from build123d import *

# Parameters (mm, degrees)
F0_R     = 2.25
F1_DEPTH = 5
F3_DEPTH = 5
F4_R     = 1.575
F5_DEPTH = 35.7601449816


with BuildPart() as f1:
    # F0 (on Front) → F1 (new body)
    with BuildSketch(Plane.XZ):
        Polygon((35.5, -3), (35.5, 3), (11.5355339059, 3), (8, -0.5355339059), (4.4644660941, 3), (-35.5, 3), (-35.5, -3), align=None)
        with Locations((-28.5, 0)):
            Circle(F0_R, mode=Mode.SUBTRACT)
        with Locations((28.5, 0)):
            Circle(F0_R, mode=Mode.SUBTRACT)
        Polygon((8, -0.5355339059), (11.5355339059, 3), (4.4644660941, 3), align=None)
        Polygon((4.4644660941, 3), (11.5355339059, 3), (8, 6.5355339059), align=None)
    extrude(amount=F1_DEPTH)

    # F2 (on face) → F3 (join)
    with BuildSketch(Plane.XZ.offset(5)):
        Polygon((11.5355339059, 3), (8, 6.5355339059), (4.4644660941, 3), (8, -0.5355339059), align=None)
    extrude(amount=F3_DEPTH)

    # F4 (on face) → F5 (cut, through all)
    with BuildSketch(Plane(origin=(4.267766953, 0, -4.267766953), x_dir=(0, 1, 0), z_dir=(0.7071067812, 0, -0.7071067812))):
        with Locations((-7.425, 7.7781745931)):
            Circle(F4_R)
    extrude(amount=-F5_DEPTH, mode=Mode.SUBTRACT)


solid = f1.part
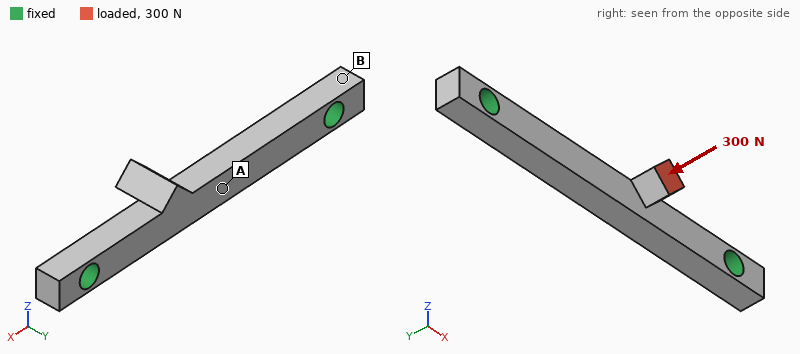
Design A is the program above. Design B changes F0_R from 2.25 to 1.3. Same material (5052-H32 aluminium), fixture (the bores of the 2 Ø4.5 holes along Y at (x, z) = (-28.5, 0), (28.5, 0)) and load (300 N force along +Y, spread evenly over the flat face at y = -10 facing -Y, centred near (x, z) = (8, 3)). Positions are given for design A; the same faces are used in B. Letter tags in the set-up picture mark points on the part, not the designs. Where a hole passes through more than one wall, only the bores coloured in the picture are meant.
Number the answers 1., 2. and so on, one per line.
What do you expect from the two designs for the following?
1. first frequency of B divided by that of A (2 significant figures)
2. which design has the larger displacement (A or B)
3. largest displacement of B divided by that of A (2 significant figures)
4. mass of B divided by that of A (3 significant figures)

1. 0.92
2. B
3. 1.1
4. 1.05
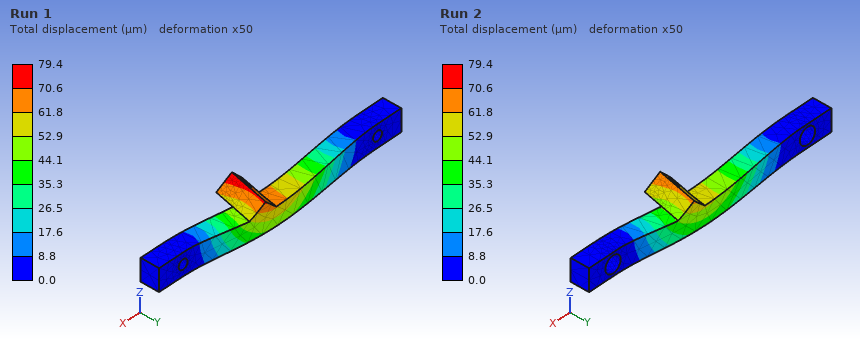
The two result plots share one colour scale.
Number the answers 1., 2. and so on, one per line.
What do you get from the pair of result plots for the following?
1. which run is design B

1. Run 1
